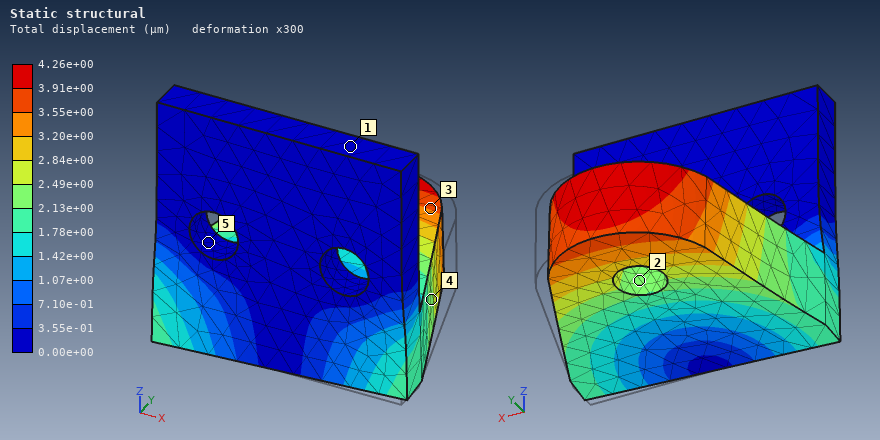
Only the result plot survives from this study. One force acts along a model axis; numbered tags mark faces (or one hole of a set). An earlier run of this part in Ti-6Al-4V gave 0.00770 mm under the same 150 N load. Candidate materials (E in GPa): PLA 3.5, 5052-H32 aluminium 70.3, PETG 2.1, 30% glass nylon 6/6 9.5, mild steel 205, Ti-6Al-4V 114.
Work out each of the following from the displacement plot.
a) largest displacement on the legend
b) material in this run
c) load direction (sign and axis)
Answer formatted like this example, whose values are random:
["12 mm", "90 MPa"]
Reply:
["4.26e+00 µm", "mild steel", "-X"]
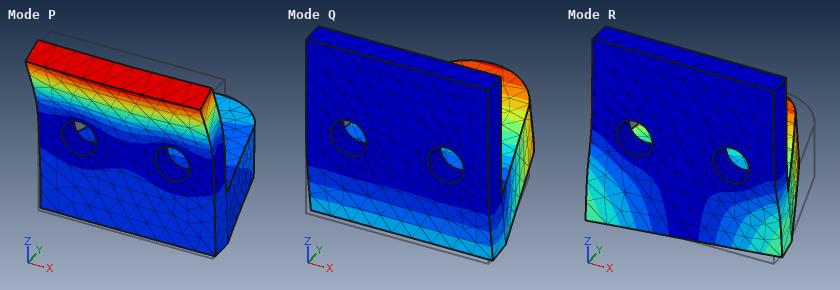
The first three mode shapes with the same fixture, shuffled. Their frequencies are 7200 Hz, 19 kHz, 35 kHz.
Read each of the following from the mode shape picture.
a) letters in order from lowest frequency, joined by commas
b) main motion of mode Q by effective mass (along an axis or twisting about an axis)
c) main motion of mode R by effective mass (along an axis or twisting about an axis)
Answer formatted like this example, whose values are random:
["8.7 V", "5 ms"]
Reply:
["Q, R, P", "along Z", "along X"]
